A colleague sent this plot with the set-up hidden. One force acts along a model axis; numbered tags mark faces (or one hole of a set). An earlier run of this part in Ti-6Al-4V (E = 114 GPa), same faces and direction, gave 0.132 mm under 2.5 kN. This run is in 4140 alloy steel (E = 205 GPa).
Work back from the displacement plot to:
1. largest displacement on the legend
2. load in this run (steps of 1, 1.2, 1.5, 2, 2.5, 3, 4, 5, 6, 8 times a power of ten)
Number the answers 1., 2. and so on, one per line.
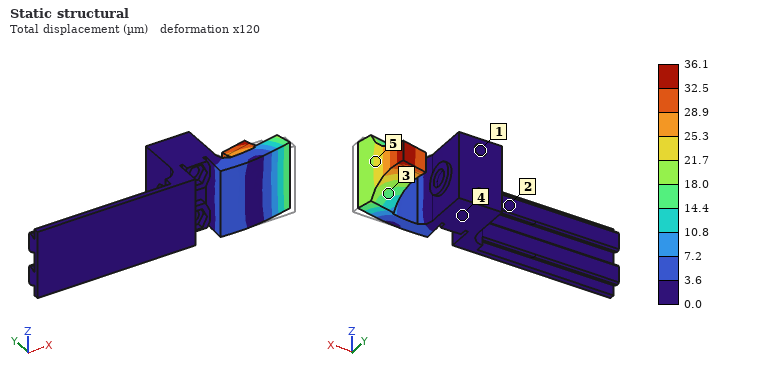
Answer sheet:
1. 36.1 µm
2. 1.2 kN
